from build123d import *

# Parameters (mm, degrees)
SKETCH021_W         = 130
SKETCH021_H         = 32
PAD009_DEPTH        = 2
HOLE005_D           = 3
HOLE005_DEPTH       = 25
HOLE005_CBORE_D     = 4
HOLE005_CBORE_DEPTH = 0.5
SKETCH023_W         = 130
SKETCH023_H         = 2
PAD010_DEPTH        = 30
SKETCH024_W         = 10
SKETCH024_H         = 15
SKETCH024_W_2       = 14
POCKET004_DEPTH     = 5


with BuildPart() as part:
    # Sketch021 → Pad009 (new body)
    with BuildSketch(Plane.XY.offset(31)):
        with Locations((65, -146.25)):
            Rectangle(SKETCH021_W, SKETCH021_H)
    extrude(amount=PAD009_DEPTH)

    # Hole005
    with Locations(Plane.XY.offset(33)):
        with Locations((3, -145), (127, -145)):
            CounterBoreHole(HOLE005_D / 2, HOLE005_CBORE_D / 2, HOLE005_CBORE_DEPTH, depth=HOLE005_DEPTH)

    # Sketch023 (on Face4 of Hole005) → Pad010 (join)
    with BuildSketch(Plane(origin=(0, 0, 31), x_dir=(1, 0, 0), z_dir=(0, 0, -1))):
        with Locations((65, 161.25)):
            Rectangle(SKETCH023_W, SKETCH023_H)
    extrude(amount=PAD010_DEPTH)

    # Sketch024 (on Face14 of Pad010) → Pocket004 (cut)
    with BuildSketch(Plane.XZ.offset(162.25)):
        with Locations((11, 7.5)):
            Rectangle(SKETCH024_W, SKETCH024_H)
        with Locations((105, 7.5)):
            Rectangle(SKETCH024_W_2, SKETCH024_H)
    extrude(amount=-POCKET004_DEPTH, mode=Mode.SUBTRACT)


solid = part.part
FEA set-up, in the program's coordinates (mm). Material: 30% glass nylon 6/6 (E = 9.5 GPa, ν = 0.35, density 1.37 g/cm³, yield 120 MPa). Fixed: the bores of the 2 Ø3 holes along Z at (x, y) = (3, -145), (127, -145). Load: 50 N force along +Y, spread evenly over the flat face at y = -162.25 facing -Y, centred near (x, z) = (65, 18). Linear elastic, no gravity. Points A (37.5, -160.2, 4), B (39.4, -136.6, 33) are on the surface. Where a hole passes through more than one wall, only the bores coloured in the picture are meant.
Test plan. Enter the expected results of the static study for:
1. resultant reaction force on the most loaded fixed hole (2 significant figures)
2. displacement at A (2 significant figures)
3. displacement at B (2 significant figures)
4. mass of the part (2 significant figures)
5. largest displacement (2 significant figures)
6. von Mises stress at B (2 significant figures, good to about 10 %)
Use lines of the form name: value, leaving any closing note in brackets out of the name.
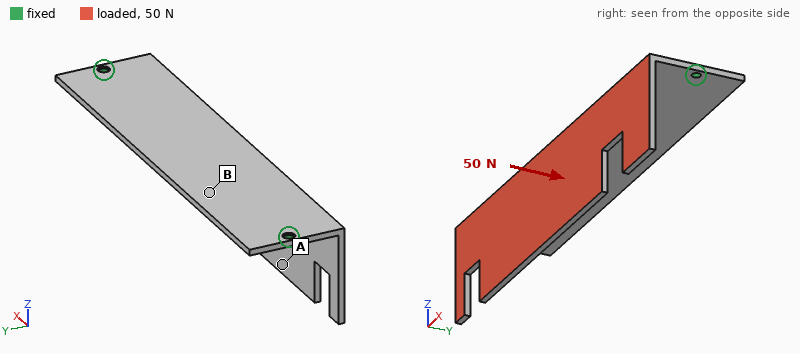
resultant reaction force on the most loaded fixed hole: 26 N
displacement at A: 1.3 mm
displacement at B: 0.48 mm
mass of the part: 21 g
largest displacement: 1.5 mm
von Mises stress at B: 5.8 MPa
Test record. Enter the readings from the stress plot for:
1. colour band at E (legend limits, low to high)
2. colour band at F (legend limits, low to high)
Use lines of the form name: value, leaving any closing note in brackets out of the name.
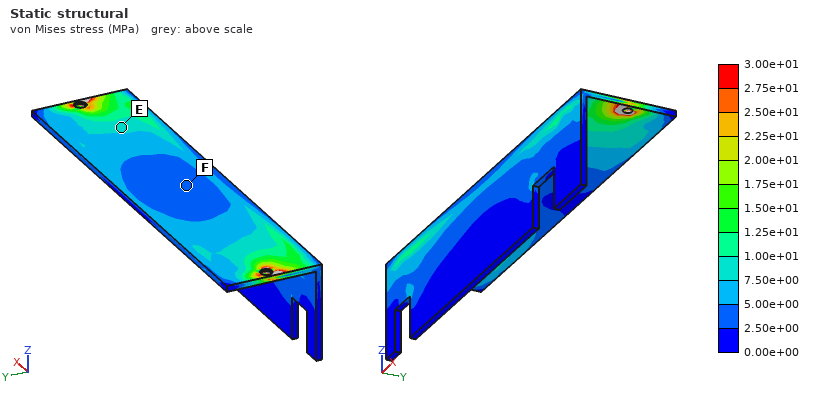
colour band at E: 7.50e+00 to 1.00e+01 MPa
colour band at F: 2.50e+00 to 5.00e+00 MPa
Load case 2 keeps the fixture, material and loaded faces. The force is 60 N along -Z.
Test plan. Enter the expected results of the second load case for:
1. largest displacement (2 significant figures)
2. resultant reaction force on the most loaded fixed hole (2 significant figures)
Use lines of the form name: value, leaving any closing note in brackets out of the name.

largest displacement: 1.3 mm
resultant reaction force on the most loaded fixed hole: 31 N
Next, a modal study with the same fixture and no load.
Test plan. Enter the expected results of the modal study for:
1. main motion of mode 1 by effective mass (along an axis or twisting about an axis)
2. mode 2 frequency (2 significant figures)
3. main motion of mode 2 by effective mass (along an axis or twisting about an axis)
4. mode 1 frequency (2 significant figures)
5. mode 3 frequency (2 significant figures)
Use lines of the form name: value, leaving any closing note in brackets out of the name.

main motion of mode 1 by effective mass: along Y
mode 2 frequency: 560 Hz
main motion of mode 2 by effective mass: along Z
mode 1 frequency: 300 Hz
mode 3 frequency: 630 Hz
